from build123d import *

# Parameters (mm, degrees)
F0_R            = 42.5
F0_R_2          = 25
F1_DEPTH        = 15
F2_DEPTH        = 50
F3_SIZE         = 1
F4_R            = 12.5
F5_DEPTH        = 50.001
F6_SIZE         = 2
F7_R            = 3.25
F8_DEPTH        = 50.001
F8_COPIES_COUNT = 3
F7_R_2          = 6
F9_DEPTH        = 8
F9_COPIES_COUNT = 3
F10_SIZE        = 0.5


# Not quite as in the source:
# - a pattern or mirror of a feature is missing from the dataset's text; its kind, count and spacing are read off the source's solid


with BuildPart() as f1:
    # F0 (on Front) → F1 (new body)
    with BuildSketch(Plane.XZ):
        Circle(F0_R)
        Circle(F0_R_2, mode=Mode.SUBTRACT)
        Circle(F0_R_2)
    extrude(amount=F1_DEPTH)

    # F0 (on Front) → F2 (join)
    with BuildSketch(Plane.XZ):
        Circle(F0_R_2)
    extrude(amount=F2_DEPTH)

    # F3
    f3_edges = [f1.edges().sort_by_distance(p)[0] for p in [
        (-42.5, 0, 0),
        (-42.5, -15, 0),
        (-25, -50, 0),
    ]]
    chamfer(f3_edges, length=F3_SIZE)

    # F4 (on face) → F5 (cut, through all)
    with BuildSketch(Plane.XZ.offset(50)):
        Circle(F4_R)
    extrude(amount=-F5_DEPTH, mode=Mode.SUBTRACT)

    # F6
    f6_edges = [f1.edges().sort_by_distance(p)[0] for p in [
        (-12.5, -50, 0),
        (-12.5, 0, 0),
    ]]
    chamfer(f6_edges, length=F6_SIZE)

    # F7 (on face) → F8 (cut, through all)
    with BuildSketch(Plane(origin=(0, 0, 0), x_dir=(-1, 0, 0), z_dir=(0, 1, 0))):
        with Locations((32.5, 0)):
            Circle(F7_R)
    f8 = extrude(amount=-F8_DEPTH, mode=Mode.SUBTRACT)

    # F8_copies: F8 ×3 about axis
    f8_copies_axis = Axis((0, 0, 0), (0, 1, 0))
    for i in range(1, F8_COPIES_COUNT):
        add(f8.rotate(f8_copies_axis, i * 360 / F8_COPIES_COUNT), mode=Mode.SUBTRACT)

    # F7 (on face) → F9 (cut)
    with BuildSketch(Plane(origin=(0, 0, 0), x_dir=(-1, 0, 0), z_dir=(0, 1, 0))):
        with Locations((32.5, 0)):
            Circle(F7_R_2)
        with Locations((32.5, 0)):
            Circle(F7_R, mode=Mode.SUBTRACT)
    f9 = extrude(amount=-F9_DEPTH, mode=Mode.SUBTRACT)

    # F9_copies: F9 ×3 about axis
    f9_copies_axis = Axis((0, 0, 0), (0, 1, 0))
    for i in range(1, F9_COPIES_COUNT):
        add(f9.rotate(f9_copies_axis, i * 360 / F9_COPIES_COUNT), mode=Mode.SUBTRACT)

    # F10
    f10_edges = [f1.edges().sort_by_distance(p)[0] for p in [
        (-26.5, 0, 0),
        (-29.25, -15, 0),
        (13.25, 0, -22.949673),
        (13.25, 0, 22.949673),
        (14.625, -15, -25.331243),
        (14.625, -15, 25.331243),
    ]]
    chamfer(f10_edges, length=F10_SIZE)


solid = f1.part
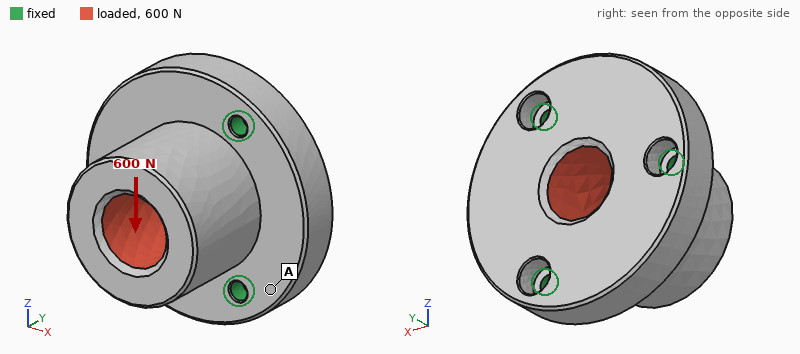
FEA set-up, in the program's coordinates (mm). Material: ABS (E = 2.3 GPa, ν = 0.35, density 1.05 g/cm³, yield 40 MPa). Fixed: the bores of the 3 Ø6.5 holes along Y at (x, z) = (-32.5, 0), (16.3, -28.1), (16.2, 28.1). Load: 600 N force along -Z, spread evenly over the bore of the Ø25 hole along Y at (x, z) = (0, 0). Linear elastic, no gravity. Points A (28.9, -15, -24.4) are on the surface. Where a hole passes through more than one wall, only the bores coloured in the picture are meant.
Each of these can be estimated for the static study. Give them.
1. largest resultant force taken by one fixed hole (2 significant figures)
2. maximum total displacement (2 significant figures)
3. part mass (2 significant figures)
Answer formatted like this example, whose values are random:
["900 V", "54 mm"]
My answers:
["240 N", "44 µm", "130 g"]
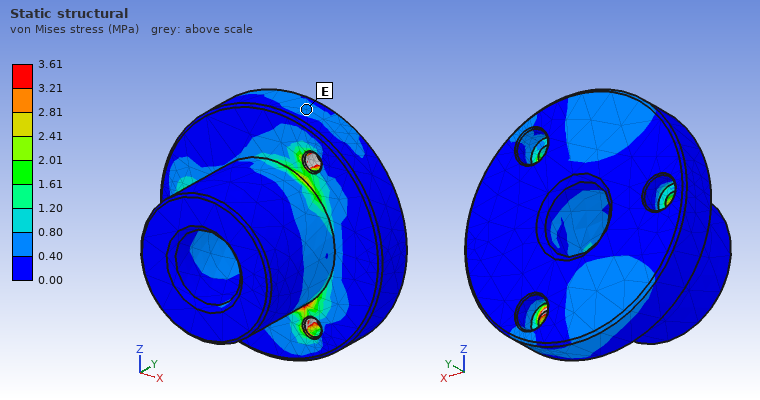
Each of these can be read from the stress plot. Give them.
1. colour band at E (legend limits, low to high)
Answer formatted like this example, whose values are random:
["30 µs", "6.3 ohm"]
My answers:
["0.40 to 0.80 MPa"]
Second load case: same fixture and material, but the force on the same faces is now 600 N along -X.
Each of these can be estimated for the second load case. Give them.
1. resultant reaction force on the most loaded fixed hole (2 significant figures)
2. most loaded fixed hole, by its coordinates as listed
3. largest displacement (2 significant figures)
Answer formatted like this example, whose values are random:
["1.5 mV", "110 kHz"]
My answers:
["250 N", "(-32.5, 0)", "45 µm"]
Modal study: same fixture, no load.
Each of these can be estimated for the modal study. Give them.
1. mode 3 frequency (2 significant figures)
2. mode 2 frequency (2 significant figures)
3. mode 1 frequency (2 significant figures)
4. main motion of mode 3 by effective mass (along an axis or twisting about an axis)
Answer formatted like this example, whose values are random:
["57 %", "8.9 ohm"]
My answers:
["2700 Hz", "2100 Hz", "2100 Hz", "along Y"]
